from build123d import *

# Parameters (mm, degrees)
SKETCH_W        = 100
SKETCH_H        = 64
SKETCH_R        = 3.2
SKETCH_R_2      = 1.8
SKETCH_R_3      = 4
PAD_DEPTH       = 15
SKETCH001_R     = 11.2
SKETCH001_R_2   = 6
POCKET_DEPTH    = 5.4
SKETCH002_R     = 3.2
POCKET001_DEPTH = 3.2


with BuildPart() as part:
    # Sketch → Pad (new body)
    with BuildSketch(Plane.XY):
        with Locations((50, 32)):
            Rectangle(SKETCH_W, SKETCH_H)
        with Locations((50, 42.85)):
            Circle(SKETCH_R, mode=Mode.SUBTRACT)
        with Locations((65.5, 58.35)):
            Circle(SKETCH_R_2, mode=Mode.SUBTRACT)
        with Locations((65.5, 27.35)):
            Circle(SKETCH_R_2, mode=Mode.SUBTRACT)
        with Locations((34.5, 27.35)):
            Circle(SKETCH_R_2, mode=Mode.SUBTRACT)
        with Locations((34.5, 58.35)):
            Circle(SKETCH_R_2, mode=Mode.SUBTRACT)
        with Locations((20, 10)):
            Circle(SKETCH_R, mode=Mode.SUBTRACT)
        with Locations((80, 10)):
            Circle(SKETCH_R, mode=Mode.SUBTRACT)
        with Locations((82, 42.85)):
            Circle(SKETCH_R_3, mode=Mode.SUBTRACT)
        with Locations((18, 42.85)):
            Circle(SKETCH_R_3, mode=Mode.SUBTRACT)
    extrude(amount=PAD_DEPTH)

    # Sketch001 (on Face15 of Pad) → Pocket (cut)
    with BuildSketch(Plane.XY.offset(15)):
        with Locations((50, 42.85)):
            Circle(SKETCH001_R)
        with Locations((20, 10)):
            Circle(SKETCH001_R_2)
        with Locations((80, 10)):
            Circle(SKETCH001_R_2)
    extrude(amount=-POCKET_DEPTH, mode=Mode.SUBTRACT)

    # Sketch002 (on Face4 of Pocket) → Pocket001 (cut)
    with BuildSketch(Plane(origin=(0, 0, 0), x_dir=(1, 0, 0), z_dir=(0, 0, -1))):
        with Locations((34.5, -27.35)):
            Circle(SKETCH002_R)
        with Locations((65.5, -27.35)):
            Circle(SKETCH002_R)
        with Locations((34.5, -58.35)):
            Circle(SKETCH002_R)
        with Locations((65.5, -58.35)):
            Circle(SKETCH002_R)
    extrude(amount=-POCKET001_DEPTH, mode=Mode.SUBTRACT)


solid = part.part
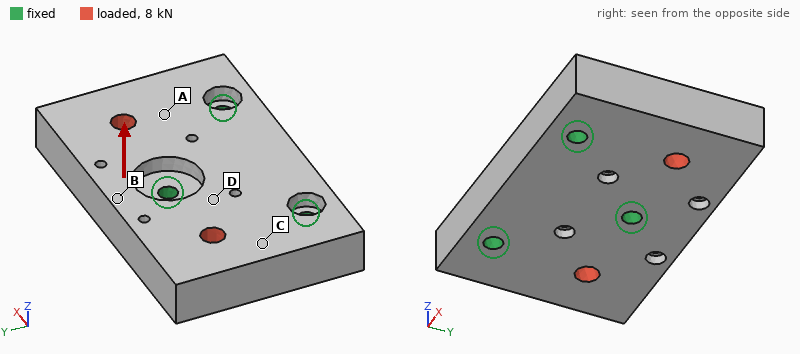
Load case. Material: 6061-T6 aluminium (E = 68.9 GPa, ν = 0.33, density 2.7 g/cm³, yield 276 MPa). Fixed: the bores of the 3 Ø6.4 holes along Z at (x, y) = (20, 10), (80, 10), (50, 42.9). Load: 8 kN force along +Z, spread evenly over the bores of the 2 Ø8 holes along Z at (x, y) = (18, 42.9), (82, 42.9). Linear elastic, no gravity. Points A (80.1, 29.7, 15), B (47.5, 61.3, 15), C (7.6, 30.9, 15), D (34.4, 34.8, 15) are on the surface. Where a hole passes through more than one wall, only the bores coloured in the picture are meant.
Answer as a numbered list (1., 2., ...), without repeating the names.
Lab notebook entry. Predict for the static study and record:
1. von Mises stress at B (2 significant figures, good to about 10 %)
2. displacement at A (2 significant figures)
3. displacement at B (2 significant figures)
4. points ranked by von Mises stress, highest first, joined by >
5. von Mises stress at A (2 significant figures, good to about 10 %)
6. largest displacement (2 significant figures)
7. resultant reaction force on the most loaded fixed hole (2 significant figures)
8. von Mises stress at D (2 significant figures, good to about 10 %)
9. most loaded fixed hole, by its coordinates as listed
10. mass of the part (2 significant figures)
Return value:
1. 50 MPa
2. 26 µm
3. 20 µm
4. B > D > A > C
5. 23 MPa
6. 88 µm
7. 5.6 kN
8. 32 MPa
9. (50, 42.9)
10. 240 g
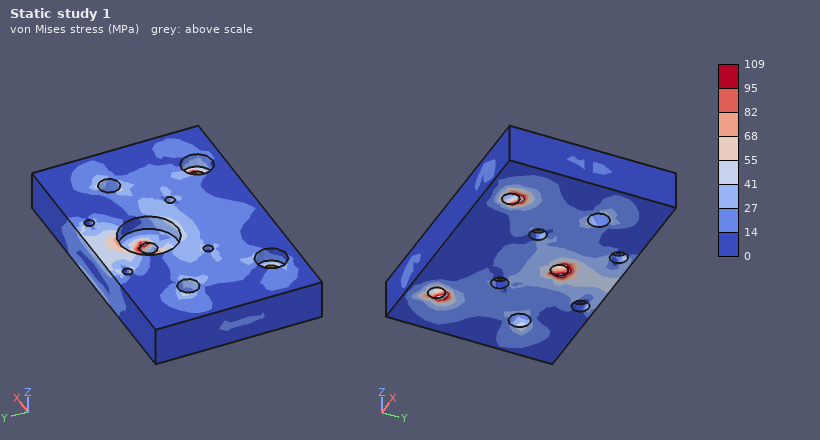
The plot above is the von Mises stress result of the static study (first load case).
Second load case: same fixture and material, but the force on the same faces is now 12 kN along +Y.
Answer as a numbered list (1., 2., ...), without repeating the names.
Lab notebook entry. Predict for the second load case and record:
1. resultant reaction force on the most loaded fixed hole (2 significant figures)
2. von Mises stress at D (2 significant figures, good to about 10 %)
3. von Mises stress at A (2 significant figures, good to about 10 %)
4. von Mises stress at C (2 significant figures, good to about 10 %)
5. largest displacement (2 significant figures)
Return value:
1. 4.3 kN
2. 7.6 MPa
3. 14 MPa
4. 7.4 MPa
5. 11 µm
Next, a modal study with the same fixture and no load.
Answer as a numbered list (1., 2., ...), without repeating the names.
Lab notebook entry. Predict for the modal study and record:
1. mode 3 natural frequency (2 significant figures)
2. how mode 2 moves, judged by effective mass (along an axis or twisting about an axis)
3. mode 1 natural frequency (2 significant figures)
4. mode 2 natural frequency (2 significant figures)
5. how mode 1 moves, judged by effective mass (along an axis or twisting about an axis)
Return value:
1. 13 kHz
2. along Z
3. 5100 Hz
4. 5600 Hz
5. twisting about Y
